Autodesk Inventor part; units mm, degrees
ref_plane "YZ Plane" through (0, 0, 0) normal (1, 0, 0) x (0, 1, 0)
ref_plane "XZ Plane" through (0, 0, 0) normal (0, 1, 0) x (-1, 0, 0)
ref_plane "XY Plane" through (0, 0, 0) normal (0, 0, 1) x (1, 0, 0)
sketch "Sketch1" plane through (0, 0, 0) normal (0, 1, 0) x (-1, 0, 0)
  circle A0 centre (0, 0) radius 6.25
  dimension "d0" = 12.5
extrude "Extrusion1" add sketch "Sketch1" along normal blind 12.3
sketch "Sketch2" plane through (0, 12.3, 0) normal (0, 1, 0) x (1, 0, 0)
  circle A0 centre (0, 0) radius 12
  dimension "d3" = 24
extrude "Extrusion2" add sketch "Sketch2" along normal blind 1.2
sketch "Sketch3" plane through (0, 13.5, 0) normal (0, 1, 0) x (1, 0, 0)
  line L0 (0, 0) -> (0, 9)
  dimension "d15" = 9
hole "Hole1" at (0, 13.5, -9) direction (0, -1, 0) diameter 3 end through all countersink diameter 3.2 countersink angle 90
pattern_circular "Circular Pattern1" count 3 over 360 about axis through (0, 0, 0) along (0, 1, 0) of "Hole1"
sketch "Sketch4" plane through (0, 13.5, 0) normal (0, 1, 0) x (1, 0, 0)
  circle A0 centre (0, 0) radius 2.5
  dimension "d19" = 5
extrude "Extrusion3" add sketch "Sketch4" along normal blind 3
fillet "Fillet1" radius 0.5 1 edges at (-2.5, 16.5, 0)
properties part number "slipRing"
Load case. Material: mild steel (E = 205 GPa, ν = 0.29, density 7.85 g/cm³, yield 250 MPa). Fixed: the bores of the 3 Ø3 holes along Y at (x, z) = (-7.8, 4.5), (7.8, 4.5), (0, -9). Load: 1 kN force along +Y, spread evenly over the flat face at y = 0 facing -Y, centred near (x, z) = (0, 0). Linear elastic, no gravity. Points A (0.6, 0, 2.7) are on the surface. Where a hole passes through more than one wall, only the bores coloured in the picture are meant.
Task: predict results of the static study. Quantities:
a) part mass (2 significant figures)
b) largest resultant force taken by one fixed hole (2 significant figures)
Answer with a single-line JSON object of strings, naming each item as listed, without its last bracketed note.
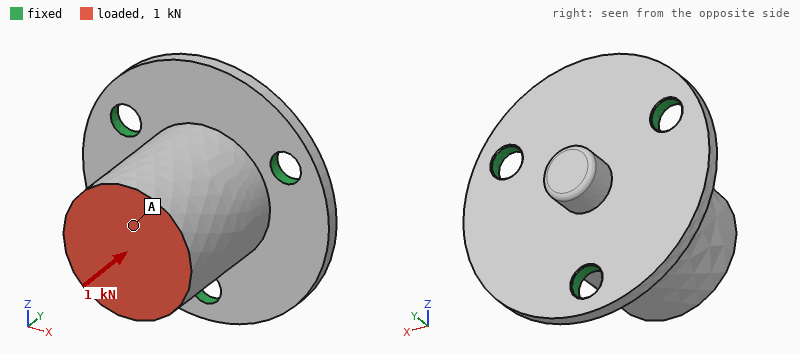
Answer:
{"part mass": "16 g", "largest resultant force taken by one fixed hole": "360 N"}
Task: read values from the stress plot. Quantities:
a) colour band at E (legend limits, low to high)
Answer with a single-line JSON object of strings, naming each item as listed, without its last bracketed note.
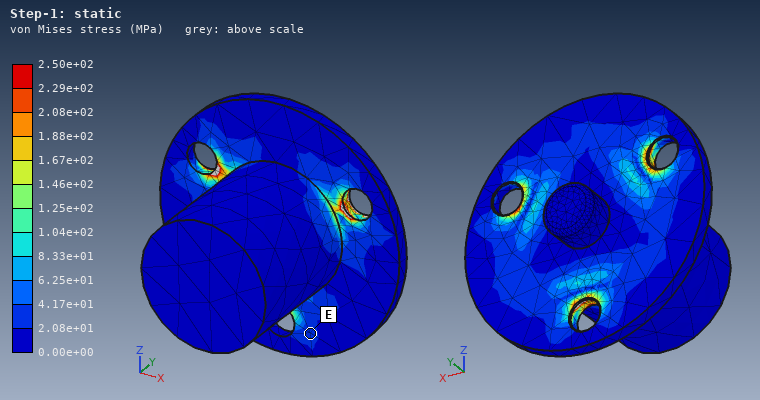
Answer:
{"colour band at E": "2.08e+01 to 4.17e+01 MPa"}
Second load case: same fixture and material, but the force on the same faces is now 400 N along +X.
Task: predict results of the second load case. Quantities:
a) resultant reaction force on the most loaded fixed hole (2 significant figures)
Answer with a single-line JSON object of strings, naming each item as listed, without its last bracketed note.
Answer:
{"resultant reaction force on the most loaded fixed hole": "440 N"}
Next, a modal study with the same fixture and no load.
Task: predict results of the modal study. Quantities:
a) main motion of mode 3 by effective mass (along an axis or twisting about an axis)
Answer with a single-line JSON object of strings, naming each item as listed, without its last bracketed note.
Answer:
{"main motion of mode 3 by effective mass": "along Y"}
